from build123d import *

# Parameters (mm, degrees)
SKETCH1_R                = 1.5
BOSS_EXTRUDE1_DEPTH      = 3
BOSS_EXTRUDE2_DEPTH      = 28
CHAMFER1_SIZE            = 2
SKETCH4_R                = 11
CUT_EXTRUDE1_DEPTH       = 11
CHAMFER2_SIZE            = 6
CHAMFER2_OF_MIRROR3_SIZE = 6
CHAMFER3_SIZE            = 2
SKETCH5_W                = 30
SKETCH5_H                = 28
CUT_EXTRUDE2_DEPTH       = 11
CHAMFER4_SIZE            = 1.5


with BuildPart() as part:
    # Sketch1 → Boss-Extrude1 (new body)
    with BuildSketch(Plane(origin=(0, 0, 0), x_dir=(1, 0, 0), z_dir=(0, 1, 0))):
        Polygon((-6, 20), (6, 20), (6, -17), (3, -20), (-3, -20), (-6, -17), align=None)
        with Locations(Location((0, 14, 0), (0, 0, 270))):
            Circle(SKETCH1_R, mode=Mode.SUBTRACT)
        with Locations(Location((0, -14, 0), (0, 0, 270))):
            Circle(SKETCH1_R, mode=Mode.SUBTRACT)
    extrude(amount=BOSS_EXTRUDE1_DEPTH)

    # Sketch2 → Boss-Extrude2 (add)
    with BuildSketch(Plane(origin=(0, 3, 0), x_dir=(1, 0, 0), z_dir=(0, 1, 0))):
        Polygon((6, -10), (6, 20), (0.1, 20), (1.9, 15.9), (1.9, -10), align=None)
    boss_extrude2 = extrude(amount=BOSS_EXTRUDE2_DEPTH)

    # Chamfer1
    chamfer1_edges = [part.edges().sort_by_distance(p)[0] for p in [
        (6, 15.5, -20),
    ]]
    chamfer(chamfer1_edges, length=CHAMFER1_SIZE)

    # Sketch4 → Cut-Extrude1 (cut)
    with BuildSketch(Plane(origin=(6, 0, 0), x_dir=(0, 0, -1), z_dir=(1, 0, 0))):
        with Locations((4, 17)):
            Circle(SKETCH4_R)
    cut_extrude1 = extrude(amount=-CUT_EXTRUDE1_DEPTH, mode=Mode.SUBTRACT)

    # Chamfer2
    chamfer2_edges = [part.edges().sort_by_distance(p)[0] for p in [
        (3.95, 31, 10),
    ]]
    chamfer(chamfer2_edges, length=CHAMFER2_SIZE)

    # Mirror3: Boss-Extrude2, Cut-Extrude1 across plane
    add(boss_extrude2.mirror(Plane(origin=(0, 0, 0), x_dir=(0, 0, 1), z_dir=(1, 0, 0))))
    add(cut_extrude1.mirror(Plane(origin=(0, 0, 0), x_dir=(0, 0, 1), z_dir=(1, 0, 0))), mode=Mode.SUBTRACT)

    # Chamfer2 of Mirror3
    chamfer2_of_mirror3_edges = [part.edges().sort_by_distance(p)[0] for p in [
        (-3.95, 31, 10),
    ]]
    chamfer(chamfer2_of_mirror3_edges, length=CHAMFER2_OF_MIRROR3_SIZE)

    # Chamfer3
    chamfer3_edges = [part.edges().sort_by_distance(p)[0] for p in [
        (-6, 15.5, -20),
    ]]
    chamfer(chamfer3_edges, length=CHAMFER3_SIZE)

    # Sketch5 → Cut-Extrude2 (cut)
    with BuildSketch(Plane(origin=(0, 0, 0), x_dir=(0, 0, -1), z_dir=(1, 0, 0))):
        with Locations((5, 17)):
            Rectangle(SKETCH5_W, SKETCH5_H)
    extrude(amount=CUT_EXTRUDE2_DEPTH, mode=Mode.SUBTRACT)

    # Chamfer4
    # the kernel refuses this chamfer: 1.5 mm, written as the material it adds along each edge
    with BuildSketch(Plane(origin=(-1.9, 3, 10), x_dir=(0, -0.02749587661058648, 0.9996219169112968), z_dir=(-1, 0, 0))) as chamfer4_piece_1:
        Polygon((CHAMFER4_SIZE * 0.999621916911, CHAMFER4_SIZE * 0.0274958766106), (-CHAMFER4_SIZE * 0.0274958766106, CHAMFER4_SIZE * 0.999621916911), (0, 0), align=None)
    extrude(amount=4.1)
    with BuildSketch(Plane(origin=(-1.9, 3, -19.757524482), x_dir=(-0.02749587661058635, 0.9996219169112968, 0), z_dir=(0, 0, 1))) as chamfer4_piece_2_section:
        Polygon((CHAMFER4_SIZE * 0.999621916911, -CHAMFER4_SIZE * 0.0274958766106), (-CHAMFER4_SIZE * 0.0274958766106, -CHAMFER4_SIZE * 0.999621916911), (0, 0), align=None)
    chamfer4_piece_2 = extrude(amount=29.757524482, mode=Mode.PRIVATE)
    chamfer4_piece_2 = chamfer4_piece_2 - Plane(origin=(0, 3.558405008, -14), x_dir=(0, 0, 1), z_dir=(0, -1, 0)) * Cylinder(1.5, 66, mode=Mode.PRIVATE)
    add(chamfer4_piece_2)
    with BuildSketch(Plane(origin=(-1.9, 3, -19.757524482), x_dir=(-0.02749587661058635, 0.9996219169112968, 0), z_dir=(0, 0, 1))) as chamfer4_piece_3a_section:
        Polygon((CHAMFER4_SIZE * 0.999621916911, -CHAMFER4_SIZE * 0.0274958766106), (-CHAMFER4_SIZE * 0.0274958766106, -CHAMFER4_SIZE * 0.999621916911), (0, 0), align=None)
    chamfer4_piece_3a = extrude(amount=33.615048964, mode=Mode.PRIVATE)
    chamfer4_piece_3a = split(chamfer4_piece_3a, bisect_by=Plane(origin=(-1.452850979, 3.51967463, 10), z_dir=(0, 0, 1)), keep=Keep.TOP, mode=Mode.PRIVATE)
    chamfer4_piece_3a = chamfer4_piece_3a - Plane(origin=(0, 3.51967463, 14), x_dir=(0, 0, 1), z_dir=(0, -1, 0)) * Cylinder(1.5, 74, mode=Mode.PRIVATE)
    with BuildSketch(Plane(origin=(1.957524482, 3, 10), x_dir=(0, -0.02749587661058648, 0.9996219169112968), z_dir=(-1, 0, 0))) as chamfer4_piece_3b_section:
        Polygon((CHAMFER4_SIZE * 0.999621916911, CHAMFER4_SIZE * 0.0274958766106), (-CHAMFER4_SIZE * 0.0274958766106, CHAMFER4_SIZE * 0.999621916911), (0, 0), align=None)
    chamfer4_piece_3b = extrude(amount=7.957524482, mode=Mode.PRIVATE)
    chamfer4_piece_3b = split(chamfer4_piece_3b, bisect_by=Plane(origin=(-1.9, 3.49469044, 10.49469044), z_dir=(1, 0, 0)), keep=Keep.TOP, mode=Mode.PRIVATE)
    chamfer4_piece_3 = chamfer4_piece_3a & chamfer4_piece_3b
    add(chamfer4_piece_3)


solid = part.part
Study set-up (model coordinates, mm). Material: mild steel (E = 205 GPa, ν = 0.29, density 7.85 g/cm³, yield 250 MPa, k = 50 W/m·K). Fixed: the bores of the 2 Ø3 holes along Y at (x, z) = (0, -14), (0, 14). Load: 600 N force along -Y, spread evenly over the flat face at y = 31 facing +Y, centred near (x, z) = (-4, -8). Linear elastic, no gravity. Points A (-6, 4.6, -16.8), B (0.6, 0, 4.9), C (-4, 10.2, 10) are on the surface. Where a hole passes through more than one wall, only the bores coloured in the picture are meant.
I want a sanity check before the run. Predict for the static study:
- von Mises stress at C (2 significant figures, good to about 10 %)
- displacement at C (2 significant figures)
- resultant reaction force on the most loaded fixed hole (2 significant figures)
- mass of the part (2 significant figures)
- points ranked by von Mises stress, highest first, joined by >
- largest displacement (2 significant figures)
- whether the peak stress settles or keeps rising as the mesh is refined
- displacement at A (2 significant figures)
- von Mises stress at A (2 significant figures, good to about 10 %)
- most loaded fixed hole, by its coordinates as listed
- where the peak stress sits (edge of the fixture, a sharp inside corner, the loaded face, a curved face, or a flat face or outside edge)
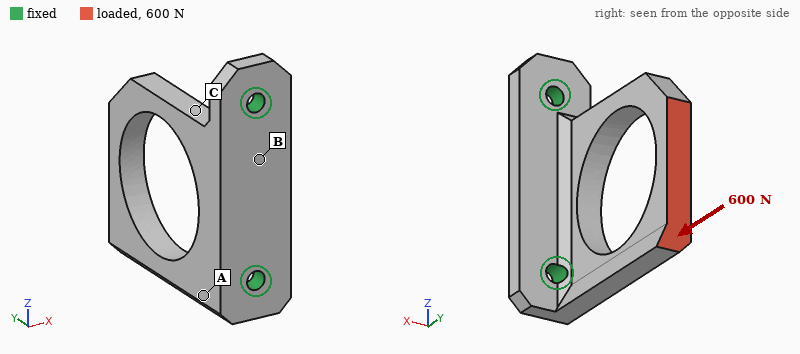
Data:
37 MPa
4.1 µm
430 N
26 g
C > A > B
15 µm
keeps rising
2.8 µm
19 MPa
(0, -14)
edge of the fixture
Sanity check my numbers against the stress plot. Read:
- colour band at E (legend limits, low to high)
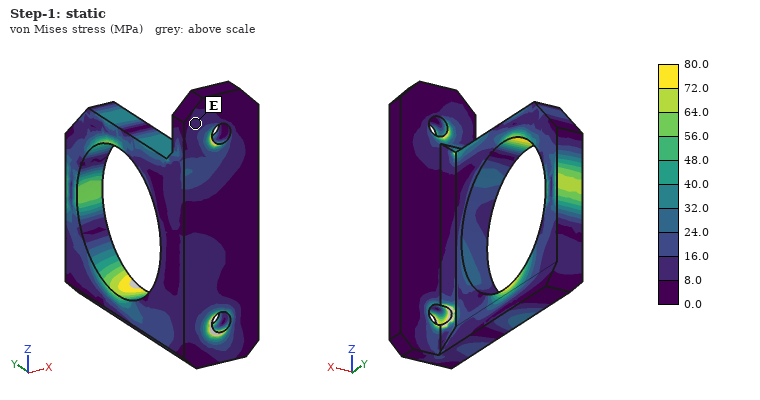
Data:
8.0 to 16.0 MPa
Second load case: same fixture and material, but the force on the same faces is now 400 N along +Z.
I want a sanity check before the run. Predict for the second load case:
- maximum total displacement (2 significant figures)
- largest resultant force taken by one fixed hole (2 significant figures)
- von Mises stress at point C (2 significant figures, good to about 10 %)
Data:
38 µm
440 N
95 MPa
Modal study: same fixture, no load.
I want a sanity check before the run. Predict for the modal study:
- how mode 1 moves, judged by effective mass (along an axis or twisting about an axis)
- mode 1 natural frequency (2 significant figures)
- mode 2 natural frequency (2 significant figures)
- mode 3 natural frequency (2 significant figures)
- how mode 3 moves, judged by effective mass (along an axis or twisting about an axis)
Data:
along X
3100 Hz
6500 Hz
8000 Hz
along Z
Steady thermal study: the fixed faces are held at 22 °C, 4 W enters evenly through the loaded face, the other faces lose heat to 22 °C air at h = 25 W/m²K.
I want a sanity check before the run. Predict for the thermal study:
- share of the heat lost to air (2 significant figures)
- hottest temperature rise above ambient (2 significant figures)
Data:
21 %
48 K
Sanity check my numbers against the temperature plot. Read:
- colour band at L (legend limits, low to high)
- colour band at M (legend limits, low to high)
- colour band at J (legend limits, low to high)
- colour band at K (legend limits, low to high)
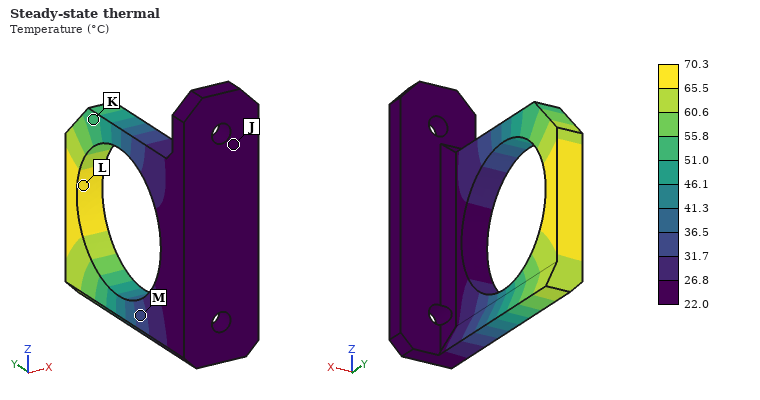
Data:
65.5 to 70.3 °C
31.7 to 36.5 °C
22.0 to 26.8 °C
51.0 to 55.8 °C
